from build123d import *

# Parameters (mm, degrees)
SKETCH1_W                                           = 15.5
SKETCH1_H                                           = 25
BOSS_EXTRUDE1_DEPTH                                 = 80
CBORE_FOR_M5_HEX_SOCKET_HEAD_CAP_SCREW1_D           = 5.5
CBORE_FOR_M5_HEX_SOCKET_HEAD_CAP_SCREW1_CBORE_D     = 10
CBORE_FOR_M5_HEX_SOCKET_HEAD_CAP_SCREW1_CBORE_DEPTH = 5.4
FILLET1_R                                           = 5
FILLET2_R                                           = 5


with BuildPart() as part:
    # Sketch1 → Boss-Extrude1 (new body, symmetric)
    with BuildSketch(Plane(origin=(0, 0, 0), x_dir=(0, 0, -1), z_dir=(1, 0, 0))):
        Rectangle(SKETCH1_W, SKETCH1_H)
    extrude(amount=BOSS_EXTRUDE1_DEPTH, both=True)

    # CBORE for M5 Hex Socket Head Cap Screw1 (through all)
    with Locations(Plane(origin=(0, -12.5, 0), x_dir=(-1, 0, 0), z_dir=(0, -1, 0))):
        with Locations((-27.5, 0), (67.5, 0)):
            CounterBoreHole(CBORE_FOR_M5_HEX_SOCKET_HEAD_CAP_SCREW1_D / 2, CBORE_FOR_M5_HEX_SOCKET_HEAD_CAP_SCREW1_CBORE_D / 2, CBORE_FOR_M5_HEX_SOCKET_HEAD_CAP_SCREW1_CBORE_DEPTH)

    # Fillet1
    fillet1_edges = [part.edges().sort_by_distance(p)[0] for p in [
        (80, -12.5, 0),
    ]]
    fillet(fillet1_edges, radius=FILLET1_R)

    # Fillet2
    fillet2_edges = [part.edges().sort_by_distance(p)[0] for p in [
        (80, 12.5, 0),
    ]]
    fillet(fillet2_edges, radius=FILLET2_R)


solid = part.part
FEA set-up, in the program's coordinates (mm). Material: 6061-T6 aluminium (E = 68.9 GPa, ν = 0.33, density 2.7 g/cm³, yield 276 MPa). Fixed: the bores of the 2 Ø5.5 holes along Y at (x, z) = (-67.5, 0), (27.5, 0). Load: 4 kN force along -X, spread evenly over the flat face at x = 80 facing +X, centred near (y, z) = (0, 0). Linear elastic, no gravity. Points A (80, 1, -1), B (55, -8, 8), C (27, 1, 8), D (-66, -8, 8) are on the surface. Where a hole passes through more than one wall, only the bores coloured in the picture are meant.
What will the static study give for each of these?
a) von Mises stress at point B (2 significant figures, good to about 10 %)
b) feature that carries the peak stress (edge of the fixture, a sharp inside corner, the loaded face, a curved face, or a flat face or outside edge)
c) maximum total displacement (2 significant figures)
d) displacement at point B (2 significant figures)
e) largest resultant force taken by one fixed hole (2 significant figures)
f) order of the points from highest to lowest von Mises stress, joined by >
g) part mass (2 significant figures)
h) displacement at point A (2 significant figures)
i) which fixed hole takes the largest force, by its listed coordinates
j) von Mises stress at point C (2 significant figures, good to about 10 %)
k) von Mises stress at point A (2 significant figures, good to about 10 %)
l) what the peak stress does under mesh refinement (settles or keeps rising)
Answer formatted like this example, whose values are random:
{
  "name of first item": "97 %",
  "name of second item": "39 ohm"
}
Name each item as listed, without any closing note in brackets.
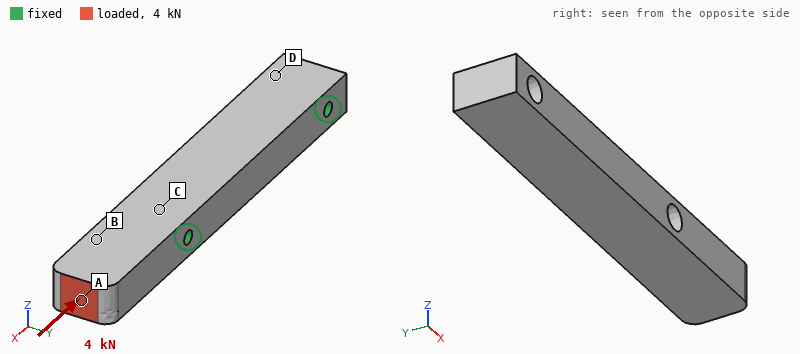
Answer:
{
  "von Mises stress at point B": "10 MPa",
  "feature that carries the peak stress": "edge of the fixture",
  "maximum total displacement": "11 µm",
  "displacement at point B": "6.0 µm",
  "largest resultant force taken by one fixed hole": "3.9 kN",
  "order of the points from highest to lowest von Mises stress, joined by >": "A > B > C > D",
  "part mass": "160 g",
  "displacement at point A": "10 µm",
  "which fixed hole takes the largest force, by its listed coordinates": "(27.5, 0)",
  "von Mises stress at point C": "5.2 MPa",
  "von Mises stress at point A": "14 MPa",
  "what the peak stress does under mesh refinement": "keeps rising"
}
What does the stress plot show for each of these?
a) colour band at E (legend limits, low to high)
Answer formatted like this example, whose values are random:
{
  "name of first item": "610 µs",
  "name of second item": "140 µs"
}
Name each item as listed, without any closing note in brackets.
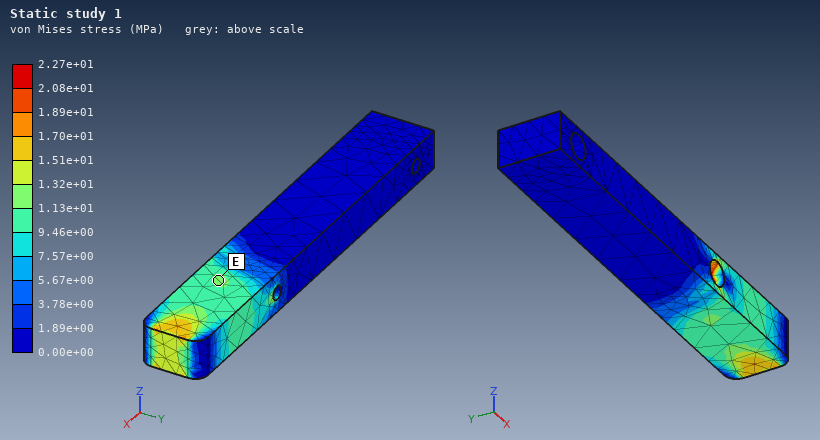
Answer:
{
  "colour band at E": "1.13e+01 to 1.32e+01 MPa"
}
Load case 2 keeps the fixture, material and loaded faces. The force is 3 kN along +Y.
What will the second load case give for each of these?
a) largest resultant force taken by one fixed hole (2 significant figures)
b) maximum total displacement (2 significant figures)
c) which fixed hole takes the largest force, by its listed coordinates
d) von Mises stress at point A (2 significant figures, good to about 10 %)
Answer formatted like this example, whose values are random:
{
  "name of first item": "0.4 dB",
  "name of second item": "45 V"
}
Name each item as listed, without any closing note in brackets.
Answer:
{
  "largest resultant force taken by one fixed hole": "3.3 kN",
  "maximum total displacement": "0.16 mm",
  "which fixed hole takes the largest force, by its listed coordinates": "(27.5, 0)",
  "von Mises stress at point A": "23 MPa"
}
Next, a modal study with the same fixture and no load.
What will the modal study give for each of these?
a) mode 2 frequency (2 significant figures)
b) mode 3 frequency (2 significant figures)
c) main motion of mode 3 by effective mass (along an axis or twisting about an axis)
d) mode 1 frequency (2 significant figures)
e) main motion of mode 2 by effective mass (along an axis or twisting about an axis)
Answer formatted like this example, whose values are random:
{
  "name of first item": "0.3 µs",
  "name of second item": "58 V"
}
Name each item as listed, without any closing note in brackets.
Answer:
{
  "mode 2 frequency": "5700 Hz",
  "mode 3 frequency": "6700 Hz",
  "main motion of mode 3 by effective mass": "along Z",
  "mode 1 frequency": "3600 Hz",
  "main motion of mode 2 by effective mass": "along Y"
}
